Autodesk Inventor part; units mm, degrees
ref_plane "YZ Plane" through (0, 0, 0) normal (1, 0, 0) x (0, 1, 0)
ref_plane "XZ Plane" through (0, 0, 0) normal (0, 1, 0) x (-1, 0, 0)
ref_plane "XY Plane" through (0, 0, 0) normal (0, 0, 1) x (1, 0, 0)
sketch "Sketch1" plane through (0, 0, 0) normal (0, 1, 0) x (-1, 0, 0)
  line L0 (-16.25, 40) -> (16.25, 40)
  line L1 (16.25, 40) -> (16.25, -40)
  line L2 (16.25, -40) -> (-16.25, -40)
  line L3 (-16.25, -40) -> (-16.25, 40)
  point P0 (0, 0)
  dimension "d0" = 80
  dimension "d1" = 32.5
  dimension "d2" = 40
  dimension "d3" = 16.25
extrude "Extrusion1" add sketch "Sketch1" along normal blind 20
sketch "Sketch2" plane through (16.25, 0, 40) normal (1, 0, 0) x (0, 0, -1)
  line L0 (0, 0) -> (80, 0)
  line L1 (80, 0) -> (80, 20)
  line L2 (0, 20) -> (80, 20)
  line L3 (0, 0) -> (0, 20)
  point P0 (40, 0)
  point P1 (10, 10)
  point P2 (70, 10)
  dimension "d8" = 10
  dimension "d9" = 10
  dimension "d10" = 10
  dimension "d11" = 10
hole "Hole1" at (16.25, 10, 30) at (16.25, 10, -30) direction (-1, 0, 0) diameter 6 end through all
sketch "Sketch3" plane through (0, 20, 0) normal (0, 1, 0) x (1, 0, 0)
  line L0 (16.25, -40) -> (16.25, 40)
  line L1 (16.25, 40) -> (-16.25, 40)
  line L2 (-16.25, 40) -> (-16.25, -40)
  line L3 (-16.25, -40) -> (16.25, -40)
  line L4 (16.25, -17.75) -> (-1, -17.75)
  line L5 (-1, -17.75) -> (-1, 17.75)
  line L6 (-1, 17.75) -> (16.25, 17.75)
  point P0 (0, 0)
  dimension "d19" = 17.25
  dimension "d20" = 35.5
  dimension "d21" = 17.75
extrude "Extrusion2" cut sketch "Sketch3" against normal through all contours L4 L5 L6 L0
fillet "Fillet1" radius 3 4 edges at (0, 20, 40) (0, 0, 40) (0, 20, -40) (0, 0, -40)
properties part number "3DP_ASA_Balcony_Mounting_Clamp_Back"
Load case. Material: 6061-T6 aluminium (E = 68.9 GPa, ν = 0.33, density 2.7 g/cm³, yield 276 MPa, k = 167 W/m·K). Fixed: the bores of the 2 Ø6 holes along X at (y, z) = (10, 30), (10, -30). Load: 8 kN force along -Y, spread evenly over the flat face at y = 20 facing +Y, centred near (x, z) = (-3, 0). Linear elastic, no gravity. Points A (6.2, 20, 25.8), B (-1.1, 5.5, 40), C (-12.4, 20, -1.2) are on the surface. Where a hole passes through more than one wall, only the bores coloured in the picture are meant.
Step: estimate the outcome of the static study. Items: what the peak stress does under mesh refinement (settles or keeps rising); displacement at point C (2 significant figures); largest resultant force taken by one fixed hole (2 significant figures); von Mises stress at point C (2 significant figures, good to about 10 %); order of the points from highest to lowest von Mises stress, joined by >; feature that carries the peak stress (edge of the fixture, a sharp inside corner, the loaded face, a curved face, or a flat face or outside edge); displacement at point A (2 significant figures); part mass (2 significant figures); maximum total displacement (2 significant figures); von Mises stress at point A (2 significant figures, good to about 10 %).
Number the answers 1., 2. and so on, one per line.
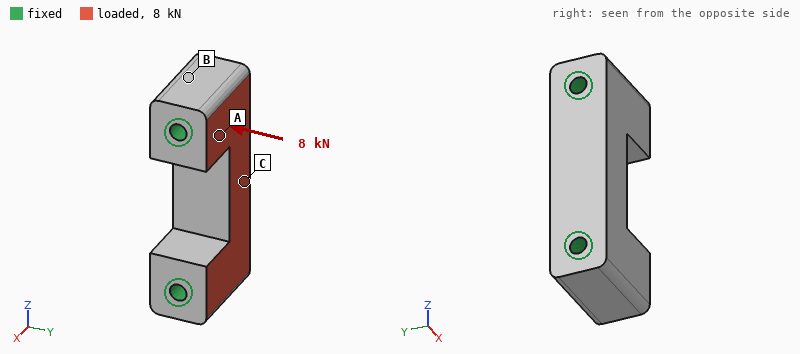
1. keeps rising
2. 9.3 µm
3. 4.0 kN
4. 14 MPa
5. C > A > B
6. edge of the fixture
7. 2.4 µm
8. 100 g
9. 9.7 µm
10. 8.3 MPa
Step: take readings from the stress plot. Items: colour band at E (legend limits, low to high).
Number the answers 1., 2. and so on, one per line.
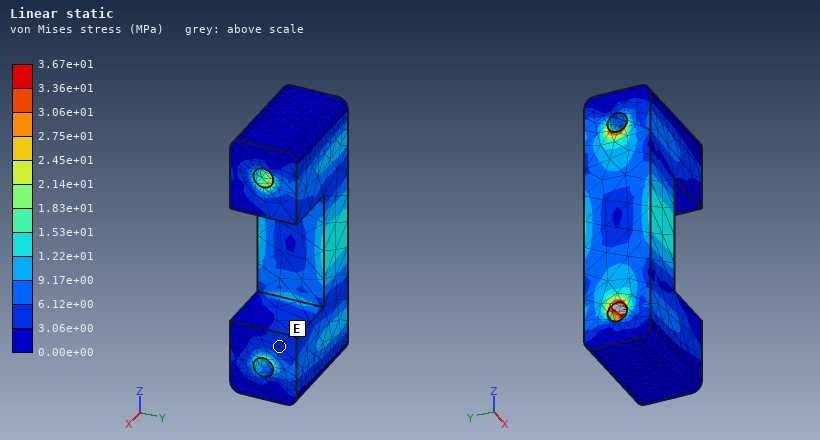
1. 3.06e+00 to 6.12e+00 MPa
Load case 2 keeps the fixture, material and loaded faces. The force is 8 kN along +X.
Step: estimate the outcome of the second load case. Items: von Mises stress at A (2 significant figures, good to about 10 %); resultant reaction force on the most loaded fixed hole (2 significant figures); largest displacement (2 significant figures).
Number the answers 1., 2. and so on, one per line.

1. 12 MPa
2. 4.0 kN
3. 15 µm
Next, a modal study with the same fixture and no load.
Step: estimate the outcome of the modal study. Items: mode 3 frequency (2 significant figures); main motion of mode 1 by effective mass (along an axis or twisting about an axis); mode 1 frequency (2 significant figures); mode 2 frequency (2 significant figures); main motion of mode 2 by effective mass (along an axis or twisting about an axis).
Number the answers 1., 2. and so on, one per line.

1. 29 kHz
2. along Y
3. 17 kHz
4. 22 kHz
5. along X
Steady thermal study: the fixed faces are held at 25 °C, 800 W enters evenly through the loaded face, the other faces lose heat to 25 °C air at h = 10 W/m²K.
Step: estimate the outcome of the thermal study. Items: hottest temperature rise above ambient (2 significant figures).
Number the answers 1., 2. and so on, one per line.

1. 72 K
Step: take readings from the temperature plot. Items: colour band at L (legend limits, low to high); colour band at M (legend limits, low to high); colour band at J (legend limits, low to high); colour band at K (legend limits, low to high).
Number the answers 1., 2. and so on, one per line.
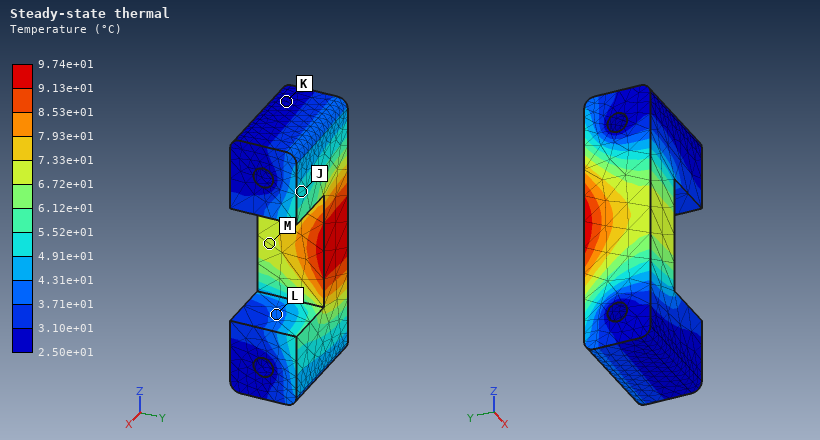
1. 3.71e+01 to 4.31e+01 °C
2. 6.72e+01 to 7.33e+01 °C
3. 4.91e+01 to 5.52e+01 °C
4. 2.50e+01 to 3.10e+01 °C
